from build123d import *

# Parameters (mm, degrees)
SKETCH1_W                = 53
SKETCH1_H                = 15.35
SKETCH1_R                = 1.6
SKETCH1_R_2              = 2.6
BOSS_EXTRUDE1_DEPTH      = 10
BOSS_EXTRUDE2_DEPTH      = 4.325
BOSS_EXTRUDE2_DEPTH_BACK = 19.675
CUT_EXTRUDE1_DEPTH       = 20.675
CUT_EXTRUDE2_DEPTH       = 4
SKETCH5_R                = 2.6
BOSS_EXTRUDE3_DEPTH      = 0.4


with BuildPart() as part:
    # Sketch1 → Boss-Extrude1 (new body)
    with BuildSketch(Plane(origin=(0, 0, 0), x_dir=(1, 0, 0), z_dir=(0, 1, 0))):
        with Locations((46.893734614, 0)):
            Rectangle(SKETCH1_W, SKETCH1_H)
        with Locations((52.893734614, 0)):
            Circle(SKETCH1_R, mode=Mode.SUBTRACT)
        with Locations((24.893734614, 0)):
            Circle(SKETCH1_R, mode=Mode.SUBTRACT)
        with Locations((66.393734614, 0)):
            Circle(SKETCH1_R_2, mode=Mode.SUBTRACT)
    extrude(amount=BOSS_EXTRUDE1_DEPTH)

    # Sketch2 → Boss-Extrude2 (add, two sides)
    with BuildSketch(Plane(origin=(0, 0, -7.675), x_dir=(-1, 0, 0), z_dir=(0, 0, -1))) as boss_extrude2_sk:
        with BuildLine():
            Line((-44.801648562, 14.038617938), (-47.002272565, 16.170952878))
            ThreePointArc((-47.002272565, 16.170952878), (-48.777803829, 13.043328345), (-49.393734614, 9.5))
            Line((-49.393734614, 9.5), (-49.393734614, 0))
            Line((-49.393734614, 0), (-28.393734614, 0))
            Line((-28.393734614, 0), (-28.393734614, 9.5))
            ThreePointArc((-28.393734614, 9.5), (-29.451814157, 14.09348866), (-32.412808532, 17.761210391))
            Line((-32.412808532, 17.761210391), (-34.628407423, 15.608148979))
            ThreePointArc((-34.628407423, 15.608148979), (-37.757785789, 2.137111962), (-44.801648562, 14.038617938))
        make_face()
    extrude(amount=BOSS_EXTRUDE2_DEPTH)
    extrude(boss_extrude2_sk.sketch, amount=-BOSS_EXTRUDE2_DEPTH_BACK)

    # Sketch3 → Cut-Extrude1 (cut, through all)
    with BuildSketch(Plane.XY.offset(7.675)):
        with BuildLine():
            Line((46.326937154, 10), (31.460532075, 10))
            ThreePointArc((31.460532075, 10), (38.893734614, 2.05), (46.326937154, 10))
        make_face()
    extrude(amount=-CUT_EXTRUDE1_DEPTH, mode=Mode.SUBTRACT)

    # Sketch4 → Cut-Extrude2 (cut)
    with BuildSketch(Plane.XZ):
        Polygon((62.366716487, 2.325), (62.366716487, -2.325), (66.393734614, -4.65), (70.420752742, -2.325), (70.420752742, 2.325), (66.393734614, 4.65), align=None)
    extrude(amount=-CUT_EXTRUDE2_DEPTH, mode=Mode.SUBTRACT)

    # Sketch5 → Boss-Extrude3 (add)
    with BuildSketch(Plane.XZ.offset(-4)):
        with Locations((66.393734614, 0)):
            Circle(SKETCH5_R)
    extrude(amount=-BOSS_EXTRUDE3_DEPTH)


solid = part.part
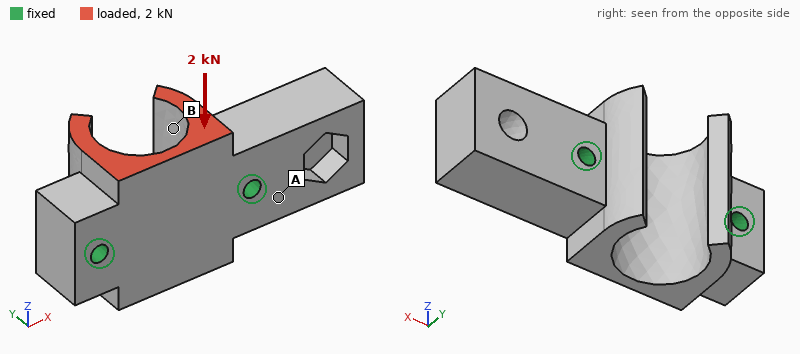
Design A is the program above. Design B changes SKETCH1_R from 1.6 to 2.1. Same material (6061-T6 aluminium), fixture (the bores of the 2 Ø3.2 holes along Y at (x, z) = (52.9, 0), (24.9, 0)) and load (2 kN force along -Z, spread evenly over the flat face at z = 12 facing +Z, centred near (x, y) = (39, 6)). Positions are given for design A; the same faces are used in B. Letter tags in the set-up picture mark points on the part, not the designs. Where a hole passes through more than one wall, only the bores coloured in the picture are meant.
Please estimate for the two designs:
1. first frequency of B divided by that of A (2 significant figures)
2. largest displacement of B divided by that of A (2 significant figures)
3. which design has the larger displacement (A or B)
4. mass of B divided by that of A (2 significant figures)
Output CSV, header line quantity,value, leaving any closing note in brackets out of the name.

quantity,value
first frequency of B divided by that of A,1.1
largest displacement of B divided by that of A,0.86
which design has the larger displacement,A
mass of B divided by that of A,0.99
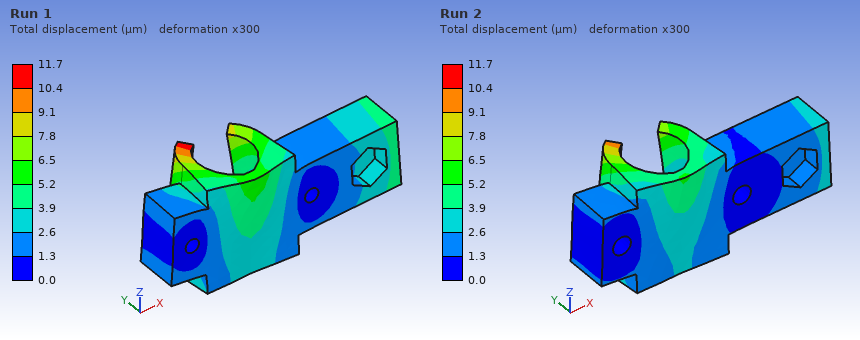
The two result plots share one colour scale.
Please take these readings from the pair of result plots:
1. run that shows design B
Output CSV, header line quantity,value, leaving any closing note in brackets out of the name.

quantity,value
run that shows design B,Run 2
